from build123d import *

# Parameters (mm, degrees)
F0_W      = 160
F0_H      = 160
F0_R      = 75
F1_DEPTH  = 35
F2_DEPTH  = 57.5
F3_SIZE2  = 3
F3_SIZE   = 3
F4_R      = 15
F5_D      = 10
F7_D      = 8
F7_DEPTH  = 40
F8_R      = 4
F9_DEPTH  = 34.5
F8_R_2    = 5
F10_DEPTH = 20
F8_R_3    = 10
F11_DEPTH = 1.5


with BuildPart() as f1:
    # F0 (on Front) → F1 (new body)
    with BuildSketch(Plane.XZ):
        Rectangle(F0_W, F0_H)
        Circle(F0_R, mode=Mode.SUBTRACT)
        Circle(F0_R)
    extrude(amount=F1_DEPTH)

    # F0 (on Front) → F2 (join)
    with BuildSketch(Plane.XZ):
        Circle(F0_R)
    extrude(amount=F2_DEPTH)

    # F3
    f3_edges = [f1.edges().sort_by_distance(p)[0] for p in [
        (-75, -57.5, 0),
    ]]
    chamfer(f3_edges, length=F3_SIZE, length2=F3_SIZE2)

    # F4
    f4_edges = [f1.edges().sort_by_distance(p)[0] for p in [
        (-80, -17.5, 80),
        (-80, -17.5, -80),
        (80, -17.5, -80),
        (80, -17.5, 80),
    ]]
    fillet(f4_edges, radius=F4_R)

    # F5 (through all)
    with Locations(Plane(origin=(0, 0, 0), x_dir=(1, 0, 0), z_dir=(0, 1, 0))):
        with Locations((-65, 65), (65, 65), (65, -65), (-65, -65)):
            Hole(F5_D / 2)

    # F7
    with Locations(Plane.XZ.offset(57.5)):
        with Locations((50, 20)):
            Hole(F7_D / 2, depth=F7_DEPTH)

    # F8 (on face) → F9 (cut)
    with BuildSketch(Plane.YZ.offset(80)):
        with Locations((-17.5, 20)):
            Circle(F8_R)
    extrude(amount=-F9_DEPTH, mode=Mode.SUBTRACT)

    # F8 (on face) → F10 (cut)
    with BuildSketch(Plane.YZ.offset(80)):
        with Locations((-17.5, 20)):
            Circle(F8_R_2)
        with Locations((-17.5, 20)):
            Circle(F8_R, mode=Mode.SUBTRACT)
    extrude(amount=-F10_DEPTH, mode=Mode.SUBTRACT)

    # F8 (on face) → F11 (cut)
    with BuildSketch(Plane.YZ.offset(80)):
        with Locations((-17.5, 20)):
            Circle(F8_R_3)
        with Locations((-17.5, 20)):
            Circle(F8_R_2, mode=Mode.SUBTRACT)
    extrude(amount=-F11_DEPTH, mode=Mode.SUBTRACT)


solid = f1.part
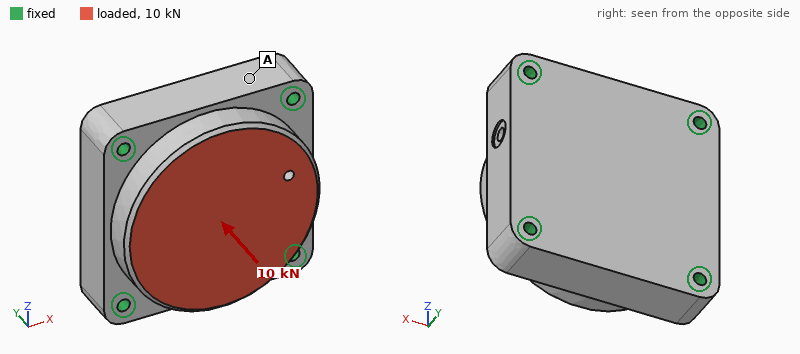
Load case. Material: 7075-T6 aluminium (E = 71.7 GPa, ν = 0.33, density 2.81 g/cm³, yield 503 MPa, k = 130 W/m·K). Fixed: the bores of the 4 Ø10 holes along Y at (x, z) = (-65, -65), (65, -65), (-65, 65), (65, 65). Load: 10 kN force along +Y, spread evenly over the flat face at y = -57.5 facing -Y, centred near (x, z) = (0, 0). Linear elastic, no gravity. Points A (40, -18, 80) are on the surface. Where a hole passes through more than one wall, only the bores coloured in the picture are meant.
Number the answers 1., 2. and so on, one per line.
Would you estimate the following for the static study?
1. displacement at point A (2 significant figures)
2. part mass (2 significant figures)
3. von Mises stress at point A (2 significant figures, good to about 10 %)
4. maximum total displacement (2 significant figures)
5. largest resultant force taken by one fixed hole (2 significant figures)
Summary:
1. 1.4 µm
2. 3.6 kg
3. 1.9 MPa
4. 3.8 µm
5. 2.6 kN
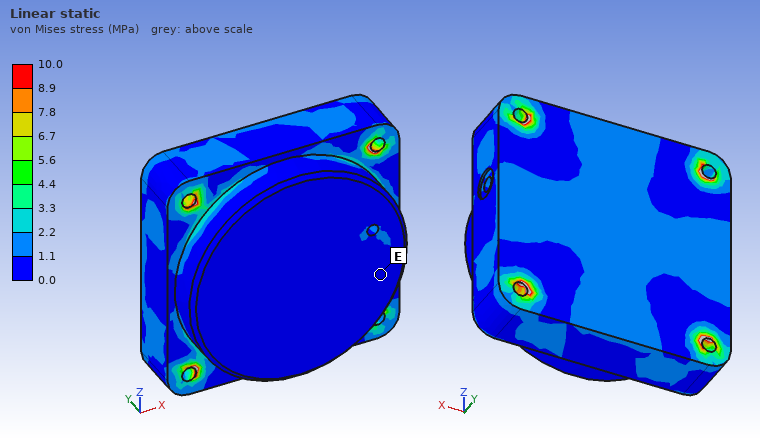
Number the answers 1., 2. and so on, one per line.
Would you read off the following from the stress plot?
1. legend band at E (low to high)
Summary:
1. 0.0 to 1.1 MPa
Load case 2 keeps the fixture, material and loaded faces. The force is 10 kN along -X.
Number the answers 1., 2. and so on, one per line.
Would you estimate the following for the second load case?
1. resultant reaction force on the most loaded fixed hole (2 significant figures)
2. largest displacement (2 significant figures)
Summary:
1. 3.1 kN
2. 4.0 µm
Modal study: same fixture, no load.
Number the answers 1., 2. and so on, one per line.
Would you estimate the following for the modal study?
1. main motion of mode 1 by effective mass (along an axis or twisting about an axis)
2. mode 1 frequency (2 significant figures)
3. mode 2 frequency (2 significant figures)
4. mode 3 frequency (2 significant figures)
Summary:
1. along Y
2. 5200 Hz
3. 7200 Hz
4. 7200 Hz
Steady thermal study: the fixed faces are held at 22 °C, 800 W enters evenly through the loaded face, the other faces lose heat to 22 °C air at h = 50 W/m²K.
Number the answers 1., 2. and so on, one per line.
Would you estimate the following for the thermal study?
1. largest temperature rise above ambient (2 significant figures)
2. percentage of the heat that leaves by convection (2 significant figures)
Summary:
1. 41 K
2. 8.4 %
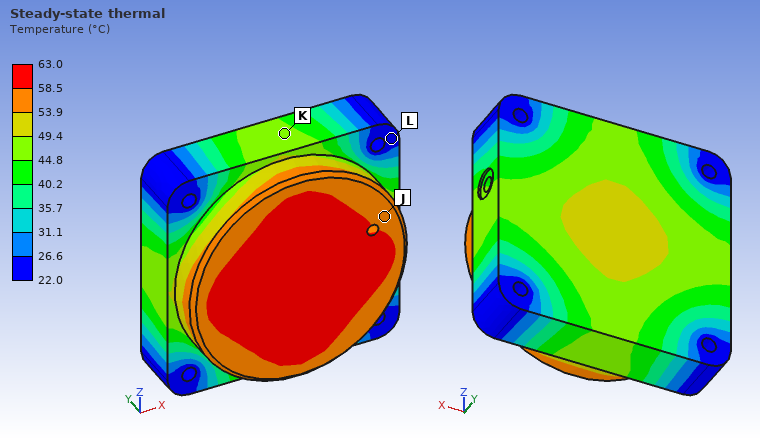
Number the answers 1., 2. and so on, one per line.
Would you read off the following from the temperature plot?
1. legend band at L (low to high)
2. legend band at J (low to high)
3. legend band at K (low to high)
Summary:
1. 22.0 to 26.6 °C
2. 53.9 to 58.5 °C
3. 44.8 to 49.4 °C
